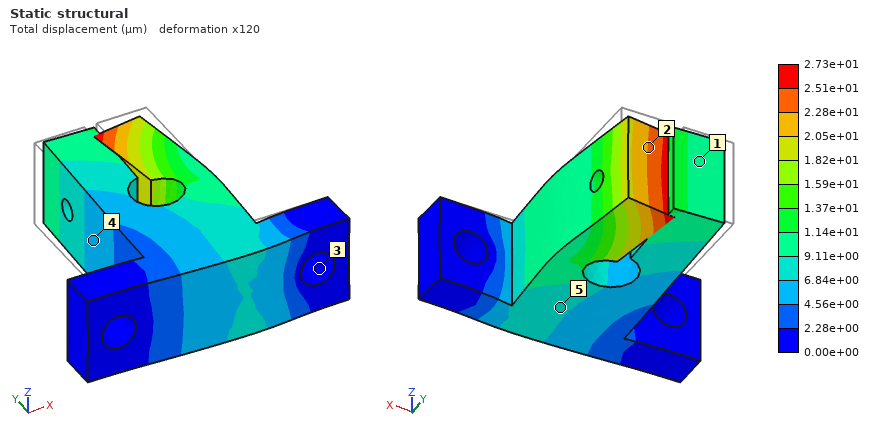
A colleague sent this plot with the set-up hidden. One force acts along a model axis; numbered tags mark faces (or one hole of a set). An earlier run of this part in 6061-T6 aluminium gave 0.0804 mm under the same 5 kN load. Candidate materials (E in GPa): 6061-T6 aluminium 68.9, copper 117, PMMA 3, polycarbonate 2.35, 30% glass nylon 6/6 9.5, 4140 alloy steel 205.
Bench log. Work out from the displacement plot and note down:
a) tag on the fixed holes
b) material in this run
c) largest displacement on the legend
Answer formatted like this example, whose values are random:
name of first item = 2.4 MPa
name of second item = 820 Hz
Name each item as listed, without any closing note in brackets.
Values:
tag on the fixed holes = 3
material in this run = 4140 alloy steel
largest displacement on the legend = 2.73e+01 µm
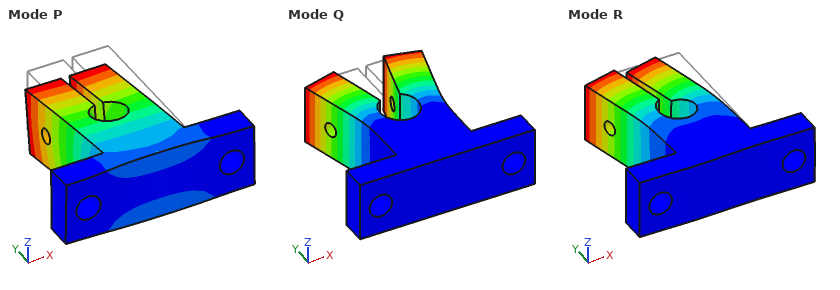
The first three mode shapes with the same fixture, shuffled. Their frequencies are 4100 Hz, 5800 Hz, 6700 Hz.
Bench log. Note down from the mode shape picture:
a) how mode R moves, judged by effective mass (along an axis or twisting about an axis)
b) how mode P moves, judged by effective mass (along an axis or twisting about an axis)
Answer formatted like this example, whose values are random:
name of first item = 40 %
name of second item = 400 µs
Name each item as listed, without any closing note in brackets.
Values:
how mode R moves, judged by effective mass = along X
how mode P moves, judged by effective mass = along Z
